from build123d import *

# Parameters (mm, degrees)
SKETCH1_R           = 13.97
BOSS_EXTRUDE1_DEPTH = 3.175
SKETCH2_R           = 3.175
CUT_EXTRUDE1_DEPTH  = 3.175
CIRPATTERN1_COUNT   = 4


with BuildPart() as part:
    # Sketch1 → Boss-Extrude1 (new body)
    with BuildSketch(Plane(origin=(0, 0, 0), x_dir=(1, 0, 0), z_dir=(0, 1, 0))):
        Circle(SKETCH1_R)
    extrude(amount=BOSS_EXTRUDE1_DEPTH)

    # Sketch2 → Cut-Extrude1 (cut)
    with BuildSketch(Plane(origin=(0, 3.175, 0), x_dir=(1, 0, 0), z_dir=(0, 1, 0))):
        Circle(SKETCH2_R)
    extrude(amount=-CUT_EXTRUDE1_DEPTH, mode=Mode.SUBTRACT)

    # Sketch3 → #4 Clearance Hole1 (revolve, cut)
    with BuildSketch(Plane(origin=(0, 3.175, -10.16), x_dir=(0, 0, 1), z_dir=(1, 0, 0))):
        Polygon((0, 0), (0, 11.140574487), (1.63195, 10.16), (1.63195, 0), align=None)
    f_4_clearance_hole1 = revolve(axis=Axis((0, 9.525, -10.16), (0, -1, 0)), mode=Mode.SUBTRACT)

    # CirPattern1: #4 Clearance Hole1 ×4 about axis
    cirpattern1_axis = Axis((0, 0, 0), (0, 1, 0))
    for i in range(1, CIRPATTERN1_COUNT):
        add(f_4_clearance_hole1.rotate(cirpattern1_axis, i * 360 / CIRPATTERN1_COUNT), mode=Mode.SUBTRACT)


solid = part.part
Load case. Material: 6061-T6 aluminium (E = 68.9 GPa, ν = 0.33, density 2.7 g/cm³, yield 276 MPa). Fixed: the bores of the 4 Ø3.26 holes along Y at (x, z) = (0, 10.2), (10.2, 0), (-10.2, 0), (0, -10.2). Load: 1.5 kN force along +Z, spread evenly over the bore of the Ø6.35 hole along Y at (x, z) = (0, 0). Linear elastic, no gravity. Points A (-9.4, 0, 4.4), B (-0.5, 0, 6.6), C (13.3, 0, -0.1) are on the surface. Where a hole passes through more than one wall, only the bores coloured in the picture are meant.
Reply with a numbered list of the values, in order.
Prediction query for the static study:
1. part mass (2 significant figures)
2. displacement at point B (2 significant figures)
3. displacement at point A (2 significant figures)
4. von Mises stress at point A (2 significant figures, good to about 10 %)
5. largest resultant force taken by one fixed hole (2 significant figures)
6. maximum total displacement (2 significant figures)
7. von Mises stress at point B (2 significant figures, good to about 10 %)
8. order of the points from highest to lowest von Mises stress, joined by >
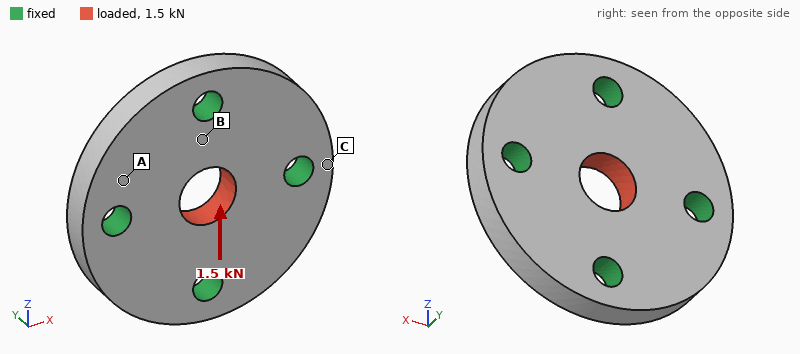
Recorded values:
1. 4.7 g
2. 0.90 µm
3. 0.57 µm
4. 7.2 MPa
5. 500 N
6. 2.7 µm
7. 29 MPa
8. B > A > C
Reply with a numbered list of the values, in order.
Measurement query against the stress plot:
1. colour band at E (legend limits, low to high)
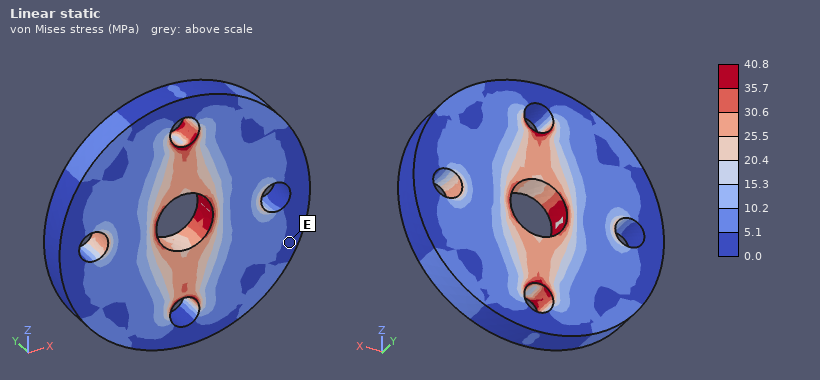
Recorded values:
1. 0.0 to 5.1 MPa
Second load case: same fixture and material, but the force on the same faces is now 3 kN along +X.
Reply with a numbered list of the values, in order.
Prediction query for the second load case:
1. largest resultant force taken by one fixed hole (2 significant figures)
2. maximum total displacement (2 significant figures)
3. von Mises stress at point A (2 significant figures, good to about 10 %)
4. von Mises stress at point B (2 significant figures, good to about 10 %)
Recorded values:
1. 990 N
2. 5.4 µm
3. 16 MPa
4. 15 MPa
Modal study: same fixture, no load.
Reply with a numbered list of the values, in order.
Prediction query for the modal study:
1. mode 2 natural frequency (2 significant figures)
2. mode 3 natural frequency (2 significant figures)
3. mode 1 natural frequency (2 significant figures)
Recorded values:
1. 53 kHz
2. 53 kHz
3. 51 kHz
